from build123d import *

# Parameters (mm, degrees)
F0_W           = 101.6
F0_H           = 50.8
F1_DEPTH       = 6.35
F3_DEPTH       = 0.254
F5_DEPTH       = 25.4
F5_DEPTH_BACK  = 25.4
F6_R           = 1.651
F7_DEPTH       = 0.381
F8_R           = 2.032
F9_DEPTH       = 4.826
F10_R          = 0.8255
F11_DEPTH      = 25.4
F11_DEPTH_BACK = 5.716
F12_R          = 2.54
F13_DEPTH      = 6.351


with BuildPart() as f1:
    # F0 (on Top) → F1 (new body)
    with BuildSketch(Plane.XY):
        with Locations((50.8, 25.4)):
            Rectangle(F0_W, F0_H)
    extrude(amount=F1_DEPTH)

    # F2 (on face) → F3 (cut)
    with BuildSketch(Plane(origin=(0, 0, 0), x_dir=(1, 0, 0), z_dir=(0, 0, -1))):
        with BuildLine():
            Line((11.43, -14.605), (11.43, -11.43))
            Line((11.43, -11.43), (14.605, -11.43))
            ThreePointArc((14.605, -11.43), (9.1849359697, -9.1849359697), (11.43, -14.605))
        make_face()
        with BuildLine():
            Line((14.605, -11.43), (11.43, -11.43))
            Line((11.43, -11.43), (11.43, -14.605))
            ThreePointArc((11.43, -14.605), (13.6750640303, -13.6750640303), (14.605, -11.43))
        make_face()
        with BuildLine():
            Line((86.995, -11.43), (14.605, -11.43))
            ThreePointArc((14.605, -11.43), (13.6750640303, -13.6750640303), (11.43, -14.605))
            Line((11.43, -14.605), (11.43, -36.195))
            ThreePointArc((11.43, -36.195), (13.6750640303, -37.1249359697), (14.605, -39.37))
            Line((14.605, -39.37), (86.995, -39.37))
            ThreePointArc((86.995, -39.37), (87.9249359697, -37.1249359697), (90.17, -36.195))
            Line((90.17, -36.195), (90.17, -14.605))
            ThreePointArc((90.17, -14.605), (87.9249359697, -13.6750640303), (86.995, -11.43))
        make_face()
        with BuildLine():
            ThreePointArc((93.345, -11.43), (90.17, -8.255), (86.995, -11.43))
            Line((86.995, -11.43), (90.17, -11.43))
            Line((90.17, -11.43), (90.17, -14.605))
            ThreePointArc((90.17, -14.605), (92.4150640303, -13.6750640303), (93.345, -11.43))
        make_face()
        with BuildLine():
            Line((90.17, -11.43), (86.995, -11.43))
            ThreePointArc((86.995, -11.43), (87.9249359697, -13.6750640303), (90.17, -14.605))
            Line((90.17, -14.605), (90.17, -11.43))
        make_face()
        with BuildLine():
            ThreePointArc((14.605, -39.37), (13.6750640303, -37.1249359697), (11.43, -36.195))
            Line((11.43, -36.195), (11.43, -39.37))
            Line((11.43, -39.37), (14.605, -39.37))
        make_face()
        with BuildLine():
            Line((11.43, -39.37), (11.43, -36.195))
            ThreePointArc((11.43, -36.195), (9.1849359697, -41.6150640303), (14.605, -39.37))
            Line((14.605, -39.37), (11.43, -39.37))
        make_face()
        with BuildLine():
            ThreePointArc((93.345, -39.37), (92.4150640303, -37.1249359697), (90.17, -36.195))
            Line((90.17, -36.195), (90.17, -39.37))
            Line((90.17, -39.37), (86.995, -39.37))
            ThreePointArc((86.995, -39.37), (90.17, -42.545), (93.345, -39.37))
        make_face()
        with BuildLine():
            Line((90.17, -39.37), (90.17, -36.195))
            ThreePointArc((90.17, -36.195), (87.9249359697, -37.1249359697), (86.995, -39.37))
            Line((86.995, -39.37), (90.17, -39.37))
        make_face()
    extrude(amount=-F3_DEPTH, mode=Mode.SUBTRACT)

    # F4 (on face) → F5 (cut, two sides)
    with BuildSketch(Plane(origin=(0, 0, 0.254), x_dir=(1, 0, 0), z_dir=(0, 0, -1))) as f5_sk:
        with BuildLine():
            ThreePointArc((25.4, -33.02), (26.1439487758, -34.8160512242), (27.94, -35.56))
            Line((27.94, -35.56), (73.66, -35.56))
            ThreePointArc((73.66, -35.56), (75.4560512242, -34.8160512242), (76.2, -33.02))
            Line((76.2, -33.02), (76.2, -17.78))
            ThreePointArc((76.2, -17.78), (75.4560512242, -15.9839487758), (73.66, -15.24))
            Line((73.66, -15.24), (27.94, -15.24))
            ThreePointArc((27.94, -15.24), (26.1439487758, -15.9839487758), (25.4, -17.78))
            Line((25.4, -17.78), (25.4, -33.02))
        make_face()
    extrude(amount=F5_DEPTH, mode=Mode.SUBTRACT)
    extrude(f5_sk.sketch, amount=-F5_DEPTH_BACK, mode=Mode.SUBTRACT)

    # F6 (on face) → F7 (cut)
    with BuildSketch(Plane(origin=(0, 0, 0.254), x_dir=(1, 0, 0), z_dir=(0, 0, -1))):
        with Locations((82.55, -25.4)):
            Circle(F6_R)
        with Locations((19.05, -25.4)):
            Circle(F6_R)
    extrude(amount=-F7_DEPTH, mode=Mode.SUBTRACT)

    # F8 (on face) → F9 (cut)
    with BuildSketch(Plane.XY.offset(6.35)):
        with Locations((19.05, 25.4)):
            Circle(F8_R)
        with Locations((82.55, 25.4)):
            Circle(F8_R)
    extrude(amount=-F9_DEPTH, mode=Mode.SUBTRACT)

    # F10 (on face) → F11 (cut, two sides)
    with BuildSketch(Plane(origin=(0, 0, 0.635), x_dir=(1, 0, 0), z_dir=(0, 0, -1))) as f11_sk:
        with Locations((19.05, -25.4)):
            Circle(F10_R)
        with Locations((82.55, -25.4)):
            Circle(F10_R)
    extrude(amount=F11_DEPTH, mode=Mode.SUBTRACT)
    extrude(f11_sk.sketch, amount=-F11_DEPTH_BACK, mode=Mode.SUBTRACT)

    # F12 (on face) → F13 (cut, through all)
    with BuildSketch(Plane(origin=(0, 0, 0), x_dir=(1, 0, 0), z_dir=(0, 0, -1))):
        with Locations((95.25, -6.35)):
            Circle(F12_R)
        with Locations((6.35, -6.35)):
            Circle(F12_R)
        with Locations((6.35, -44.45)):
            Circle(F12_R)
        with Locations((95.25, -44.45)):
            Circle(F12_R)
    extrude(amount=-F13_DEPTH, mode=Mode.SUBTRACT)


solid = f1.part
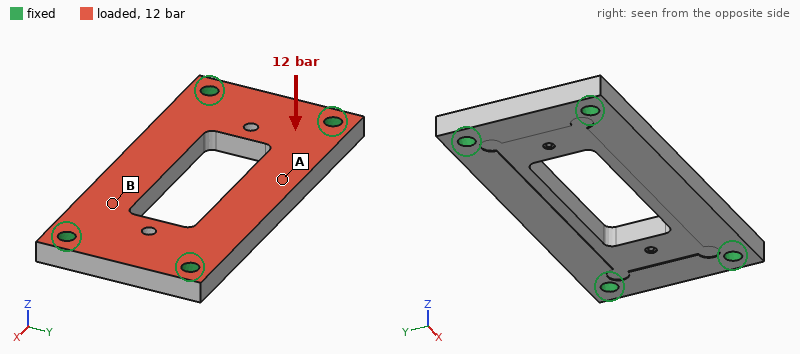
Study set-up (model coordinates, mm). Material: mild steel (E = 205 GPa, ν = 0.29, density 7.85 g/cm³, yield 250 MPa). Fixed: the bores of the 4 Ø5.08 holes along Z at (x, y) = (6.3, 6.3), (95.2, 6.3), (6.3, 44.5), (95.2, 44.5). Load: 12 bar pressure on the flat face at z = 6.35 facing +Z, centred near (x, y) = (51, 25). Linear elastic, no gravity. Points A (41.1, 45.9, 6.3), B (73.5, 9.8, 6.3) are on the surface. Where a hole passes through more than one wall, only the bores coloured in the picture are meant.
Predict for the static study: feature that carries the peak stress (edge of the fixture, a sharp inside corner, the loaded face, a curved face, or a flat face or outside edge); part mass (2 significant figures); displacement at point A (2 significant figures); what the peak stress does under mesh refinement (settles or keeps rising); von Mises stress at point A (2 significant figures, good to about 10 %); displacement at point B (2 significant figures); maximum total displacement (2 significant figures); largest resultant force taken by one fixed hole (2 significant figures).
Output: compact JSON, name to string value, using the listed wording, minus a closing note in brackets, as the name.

{"feature that carries the peak stress": "edge of the fixture", "part mass": "200 g", "displacement at point A": "39 µm", "what the peak stress does under mesh refinement": "keeps rising", "von Mises stress at point A": "46 MPa", "displacement at point B": "25 µm", "maximum total displacement": "46 µm", "largest resultant force taken by one fixed hole": "1.2 kN"}
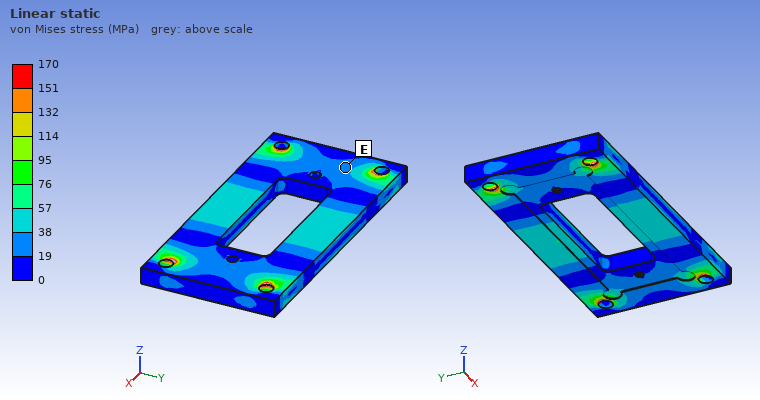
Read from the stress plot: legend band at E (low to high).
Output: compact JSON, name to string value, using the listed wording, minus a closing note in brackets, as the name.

{"legend band at E": "19 to 38 MPa"}
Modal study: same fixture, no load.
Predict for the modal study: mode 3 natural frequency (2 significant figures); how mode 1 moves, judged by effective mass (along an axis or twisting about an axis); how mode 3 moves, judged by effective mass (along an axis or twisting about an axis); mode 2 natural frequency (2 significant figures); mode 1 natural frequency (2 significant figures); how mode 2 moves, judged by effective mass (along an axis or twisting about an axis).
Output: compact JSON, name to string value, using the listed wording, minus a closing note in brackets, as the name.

{"mode 3 natural frequency": "10 kHz", "how mode 1 moves, judged by effective mass": "along Z", "how mode 3 moves, judged by effective mass": "twisting about Y", "mode 2 natural frequency": "5000 Hz", "mode 1 natural frequency": "4400 Hz", "how mode 2 moves, judged by effective mass": "twisting about X"}
